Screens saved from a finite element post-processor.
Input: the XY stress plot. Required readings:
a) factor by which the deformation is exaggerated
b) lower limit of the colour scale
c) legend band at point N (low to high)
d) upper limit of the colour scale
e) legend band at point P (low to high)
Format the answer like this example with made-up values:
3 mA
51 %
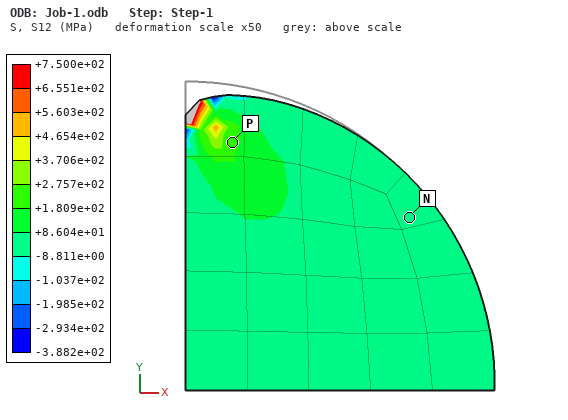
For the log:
50
-3.882e+02 MPa
-8.811e+00 to +8.604e+01 MPa
+7.500e+02 MPa
+1.809e+02 to +2.757e+02 MPa
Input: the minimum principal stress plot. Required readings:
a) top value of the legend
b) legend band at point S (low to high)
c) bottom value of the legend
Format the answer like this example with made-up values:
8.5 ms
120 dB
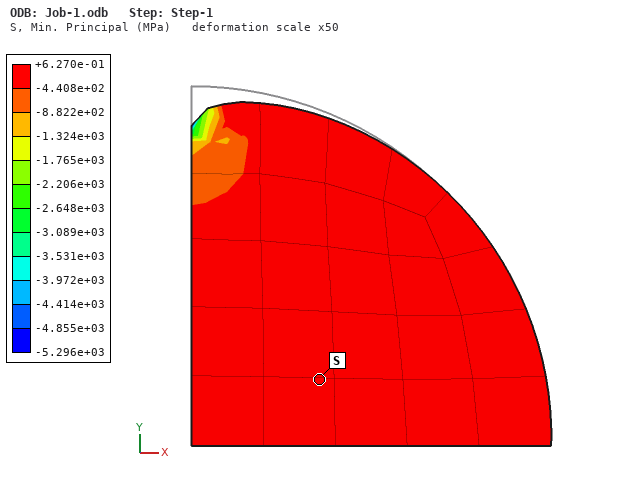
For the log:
+6.270e-01 MPa
-4.408e+02 to +6.270e-01 MPa
-5.296e+03 MPa
